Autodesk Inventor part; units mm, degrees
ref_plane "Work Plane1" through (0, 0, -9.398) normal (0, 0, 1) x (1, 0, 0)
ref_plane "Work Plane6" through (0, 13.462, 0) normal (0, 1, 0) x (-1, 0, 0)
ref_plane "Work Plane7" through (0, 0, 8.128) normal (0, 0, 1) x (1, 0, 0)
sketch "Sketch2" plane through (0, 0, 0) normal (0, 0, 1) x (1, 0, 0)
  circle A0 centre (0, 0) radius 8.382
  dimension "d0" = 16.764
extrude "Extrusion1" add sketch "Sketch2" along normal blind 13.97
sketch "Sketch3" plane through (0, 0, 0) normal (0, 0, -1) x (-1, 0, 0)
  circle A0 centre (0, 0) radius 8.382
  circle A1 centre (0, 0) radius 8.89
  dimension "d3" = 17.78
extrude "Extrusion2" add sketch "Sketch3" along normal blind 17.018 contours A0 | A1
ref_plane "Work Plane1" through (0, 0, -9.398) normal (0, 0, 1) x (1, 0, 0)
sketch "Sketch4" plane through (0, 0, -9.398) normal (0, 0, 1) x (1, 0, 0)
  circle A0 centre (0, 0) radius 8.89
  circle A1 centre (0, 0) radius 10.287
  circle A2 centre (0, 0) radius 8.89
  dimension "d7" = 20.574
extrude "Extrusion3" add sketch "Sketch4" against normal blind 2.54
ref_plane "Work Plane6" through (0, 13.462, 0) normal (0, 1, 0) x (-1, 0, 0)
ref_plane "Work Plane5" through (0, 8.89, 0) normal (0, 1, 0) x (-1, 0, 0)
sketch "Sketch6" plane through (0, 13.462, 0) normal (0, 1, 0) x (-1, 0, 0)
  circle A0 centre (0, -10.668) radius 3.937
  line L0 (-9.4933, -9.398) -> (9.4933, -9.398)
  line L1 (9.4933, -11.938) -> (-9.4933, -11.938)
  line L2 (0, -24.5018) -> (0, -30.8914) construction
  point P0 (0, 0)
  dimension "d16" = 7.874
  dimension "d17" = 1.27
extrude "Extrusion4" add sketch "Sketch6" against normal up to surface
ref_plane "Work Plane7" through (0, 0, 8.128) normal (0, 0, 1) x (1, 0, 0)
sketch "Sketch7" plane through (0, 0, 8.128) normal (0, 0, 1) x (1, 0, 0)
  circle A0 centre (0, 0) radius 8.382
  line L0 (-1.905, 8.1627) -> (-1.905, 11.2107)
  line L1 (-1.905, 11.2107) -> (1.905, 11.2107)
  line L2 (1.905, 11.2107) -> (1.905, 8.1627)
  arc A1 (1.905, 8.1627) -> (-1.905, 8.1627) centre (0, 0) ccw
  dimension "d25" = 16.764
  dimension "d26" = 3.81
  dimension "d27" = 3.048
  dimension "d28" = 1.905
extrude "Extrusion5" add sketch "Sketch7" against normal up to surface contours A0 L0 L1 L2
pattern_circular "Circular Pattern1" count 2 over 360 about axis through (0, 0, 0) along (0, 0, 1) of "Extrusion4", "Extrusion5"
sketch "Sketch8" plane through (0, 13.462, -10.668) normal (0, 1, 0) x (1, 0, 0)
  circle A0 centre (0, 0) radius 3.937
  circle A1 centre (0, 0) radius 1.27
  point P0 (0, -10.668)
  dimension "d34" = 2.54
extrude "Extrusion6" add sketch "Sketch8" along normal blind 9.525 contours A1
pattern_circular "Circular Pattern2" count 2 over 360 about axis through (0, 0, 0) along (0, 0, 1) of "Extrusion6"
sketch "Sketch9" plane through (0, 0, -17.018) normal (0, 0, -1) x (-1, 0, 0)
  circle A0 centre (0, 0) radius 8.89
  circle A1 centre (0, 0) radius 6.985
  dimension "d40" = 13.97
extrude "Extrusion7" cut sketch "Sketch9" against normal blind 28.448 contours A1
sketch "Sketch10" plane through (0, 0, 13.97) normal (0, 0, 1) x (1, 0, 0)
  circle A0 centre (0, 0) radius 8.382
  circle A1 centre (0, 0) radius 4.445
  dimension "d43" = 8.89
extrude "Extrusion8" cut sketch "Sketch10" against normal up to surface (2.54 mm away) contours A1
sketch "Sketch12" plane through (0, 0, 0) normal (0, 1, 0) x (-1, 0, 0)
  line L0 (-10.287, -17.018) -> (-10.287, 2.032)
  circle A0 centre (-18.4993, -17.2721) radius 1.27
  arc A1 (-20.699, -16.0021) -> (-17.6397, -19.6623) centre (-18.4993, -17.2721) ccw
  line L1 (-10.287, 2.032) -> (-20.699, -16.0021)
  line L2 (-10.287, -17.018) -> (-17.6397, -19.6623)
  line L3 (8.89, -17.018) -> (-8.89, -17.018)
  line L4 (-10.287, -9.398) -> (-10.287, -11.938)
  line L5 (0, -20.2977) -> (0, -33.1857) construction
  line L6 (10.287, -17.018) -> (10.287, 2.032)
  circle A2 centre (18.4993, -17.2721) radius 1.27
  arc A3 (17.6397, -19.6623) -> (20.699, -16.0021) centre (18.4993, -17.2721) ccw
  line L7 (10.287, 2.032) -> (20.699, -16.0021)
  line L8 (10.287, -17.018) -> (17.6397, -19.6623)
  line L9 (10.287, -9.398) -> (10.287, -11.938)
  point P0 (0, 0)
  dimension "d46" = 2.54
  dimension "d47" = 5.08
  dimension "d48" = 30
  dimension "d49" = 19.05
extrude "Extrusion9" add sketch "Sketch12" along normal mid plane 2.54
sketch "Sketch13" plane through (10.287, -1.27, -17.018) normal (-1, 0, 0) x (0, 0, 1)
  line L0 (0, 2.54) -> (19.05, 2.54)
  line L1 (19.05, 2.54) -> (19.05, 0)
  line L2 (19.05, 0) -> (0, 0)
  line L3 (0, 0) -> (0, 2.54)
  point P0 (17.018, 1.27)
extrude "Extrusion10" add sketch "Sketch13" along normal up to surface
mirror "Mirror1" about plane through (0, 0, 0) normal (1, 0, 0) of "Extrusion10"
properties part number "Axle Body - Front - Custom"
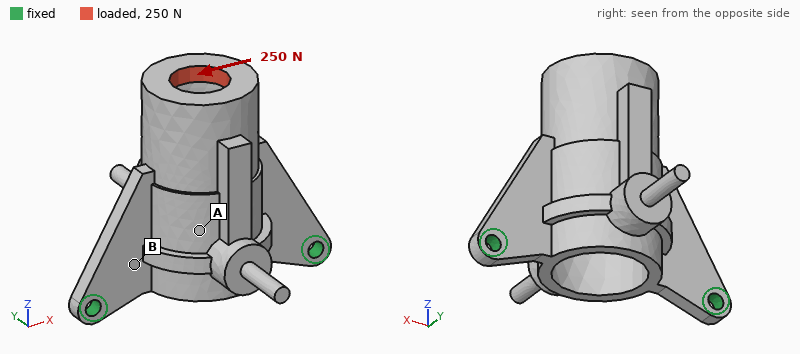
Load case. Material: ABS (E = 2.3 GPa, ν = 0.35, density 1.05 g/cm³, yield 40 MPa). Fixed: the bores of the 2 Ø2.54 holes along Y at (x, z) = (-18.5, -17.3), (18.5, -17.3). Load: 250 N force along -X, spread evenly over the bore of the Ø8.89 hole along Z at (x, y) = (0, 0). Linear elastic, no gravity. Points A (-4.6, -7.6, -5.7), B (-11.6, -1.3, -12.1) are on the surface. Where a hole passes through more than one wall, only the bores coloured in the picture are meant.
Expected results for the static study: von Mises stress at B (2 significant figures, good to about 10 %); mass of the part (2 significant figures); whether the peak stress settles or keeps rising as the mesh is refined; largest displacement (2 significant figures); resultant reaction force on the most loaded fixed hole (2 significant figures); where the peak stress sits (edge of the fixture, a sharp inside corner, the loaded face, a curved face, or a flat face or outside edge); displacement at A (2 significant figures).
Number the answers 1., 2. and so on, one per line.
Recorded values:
1. 9.5 MPa
2. 4.8 g
3. keeps rising
4. 0.44 mm
5. 240 N
6. edge of the fixture
7. 0.088 mm
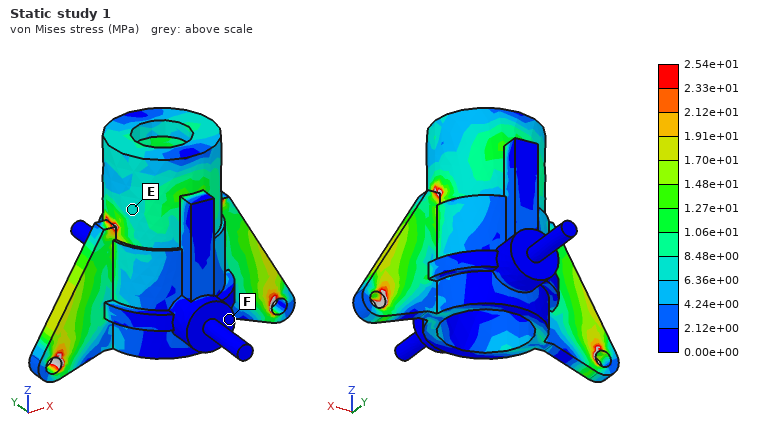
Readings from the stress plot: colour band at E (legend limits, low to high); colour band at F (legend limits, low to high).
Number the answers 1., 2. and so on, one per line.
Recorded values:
1. 6.36e+00 to 8.48e+00 MPa
2. 0.00e+00 to 2.12e+00 MPa
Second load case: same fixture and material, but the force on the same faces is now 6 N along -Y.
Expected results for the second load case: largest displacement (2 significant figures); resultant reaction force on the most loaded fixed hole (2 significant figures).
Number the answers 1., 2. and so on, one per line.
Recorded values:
1. 0.69 mm
2. 3.0 N
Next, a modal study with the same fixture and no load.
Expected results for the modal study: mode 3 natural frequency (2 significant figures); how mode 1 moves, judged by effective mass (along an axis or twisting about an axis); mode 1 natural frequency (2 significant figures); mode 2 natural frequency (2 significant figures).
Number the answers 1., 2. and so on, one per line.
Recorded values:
1. 2400 Hz
2. along Y
3. 400 Hz
4. 2300 Hz
